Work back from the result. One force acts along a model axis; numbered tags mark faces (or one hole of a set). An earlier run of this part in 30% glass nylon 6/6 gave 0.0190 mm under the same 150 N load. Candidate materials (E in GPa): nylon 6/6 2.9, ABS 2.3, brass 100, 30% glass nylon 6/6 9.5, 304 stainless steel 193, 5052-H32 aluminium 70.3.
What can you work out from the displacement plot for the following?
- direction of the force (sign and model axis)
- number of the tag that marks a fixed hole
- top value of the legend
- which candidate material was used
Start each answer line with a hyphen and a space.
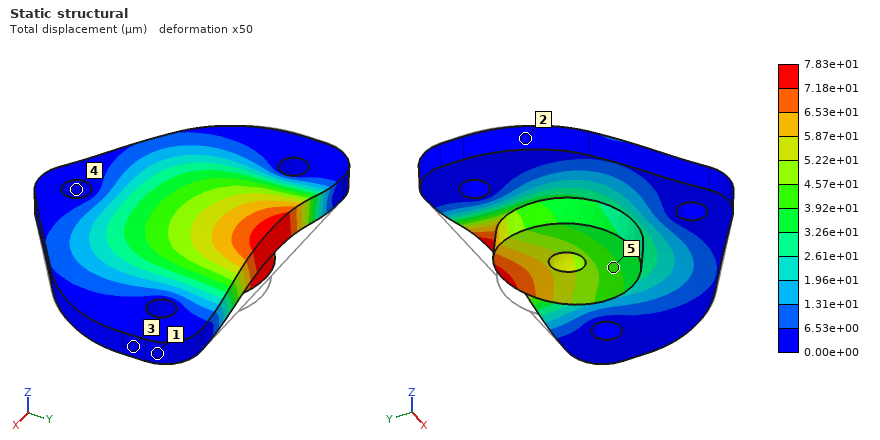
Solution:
- +Z
- 4
- 7.83e+01 µm
- ABS
